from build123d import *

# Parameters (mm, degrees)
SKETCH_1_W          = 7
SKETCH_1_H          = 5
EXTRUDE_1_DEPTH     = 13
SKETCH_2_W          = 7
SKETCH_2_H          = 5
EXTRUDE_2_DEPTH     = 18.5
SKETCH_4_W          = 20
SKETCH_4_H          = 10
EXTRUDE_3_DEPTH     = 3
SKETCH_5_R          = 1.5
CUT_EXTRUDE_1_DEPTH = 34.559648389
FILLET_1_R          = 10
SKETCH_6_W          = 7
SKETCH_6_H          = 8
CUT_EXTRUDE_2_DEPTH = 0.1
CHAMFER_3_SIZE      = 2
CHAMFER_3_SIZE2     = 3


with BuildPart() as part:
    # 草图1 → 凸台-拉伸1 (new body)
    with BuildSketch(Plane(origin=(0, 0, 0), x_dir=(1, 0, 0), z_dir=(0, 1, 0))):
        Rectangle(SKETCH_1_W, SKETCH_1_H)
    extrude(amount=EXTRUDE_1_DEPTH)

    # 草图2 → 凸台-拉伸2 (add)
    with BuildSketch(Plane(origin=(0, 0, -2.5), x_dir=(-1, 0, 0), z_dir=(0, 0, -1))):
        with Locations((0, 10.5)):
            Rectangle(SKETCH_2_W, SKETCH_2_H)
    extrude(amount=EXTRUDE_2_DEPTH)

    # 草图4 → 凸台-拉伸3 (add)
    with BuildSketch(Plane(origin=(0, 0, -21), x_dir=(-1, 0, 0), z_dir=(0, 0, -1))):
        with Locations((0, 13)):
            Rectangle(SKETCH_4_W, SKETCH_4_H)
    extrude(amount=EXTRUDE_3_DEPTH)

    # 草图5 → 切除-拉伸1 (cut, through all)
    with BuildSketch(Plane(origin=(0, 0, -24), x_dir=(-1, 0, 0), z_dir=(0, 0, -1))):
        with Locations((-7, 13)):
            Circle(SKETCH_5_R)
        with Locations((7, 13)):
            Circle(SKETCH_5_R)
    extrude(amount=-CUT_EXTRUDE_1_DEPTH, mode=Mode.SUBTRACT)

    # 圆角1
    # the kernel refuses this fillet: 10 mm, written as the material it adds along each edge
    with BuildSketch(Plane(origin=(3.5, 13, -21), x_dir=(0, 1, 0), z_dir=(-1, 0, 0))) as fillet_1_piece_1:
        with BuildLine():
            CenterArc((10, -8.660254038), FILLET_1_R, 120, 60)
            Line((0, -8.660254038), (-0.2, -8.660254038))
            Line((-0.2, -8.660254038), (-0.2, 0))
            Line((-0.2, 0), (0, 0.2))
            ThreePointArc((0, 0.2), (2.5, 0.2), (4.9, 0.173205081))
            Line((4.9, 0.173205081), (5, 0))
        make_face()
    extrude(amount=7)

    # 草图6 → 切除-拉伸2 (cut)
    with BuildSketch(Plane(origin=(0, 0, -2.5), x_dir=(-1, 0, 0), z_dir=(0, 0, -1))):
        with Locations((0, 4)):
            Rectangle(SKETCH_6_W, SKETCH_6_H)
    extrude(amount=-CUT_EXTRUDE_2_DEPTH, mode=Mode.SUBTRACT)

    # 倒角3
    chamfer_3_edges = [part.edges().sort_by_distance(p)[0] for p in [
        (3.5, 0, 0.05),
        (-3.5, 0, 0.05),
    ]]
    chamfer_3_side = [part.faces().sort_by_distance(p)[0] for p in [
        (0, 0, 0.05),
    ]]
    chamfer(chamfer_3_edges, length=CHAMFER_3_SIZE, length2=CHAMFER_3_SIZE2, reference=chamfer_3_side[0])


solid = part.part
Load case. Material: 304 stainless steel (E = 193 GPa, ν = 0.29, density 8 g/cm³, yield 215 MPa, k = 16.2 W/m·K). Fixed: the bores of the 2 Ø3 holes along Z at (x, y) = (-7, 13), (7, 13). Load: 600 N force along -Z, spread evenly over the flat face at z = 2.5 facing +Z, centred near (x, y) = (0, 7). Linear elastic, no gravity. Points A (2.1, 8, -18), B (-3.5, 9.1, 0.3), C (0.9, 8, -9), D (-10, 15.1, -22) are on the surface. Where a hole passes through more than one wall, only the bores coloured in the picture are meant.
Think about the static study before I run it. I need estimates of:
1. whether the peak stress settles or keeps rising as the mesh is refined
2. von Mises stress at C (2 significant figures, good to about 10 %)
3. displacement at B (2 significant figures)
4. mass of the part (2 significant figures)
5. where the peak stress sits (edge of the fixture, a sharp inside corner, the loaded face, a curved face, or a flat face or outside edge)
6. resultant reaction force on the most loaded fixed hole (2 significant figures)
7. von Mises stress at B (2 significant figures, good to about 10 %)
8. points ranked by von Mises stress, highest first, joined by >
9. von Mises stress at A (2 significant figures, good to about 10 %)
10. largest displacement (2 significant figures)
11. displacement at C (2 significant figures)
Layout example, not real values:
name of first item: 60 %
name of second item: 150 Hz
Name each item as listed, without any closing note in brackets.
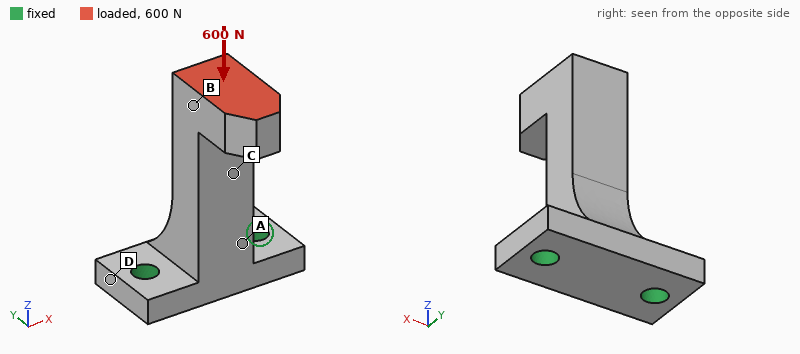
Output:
whether the peak stress settles or keeps rising as the mesh is refined: keeps rising
von Mises stress at C: 91 MPa
displacement at B: 52 µm
mass of the part: 14 g
where the peak stress sits: edge of the fixture
resultant reaction force on the most loaded fixed hole: 320 N
von Mises stress at B: 31 MPa
points ranked by von Mises stress, highest first, joined by >: C > A > B > D
von Mises stress at A: 67 MPa
largest displacement: 77 µm
displacement at C: 24 µm
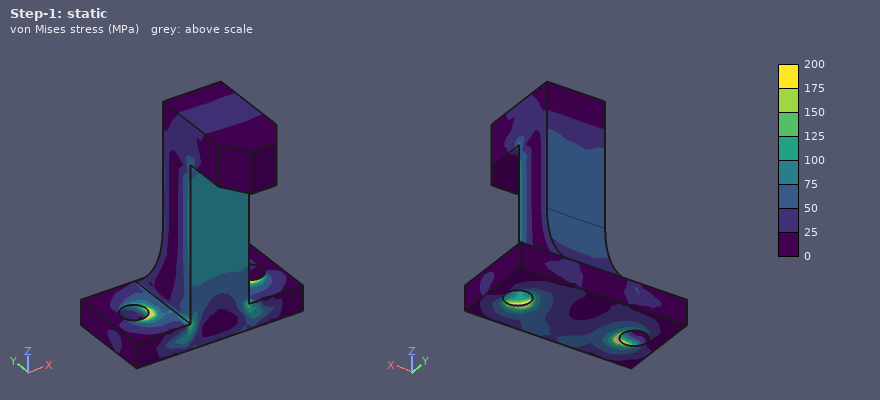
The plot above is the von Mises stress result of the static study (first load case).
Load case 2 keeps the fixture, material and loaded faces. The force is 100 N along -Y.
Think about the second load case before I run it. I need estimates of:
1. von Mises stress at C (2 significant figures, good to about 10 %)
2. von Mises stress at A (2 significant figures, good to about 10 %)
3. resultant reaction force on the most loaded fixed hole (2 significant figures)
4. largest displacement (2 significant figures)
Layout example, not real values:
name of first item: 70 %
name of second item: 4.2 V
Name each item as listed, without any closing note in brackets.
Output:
von Mises stress at C: 39 MPa
von Mises stress at A: 42 MPa
resultant reaction force on the most loaded fixed hole: 53 N
largest displacement: 46 µm
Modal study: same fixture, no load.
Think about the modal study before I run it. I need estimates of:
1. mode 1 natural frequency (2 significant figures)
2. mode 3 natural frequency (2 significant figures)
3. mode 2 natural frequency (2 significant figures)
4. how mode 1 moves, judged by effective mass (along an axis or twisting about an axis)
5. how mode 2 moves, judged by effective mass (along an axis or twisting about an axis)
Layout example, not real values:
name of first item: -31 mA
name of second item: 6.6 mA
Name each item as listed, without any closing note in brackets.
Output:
mode 1 natural frequency: 4200 Hz
mode 3 natural frequency: 16 kHz
mode 2 natural frequency: 6000 Hz
how mode 1 moves, judged by effective mass: along Y
how mode 2 moves, judged by effective mass: along X
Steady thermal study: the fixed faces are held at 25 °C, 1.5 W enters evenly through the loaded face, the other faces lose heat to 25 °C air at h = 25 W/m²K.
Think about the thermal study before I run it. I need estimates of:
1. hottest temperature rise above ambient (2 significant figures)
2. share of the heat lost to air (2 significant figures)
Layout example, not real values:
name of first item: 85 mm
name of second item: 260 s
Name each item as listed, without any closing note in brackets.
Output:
hottest temperature rise above ambient: 51 K
share of the heat lost to air: 35 %
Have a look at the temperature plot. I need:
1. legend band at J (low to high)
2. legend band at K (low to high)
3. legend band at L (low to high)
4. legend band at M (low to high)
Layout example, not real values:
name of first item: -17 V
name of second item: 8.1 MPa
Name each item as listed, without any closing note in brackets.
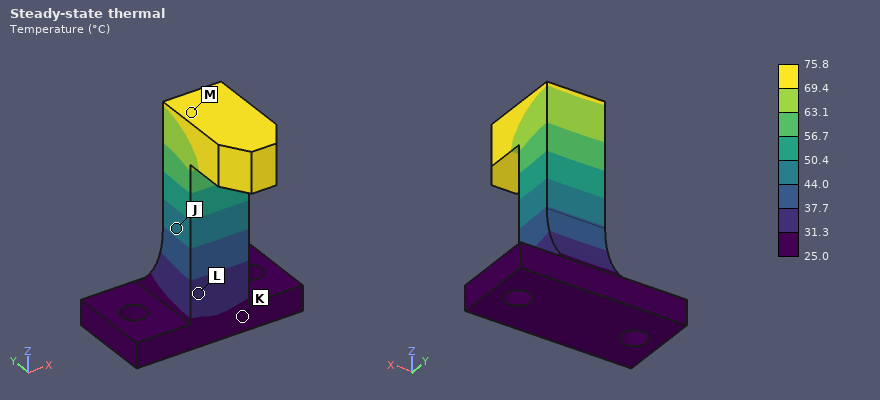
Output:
legend band at J: 44.0 to 50.4 °C
legend band at K: 25.0 to 31.3 °C
legend band at L: 31.3 to 37.7 °C
legend band at M: 69.4 to 75.8 °C
